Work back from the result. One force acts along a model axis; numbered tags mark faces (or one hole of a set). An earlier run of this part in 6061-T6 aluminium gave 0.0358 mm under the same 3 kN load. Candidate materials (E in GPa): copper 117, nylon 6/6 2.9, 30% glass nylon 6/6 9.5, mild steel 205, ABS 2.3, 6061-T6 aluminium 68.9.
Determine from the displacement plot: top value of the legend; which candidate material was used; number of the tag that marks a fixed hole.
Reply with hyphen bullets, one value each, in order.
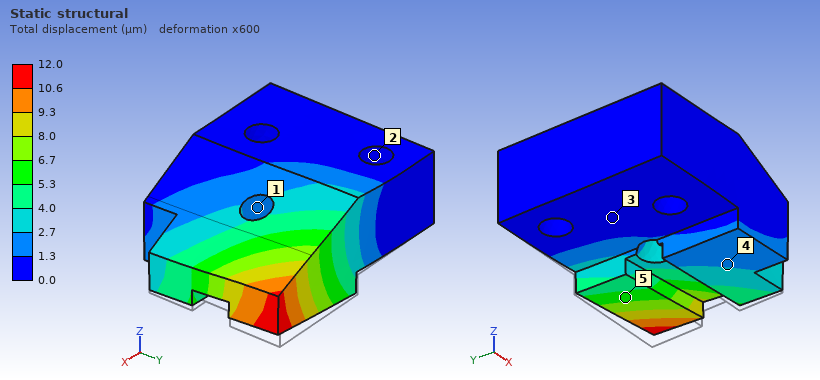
- 12.0 µm
- mild steel
- 2
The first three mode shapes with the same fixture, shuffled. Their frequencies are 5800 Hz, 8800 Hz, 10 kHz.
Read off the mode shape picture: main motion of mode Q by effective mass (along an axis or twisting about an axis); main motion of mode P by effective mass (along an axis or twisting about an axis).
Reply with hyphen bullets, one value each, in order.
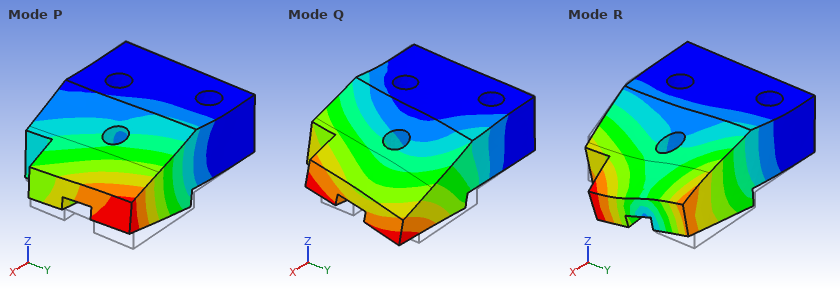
- along Y
- along Z
